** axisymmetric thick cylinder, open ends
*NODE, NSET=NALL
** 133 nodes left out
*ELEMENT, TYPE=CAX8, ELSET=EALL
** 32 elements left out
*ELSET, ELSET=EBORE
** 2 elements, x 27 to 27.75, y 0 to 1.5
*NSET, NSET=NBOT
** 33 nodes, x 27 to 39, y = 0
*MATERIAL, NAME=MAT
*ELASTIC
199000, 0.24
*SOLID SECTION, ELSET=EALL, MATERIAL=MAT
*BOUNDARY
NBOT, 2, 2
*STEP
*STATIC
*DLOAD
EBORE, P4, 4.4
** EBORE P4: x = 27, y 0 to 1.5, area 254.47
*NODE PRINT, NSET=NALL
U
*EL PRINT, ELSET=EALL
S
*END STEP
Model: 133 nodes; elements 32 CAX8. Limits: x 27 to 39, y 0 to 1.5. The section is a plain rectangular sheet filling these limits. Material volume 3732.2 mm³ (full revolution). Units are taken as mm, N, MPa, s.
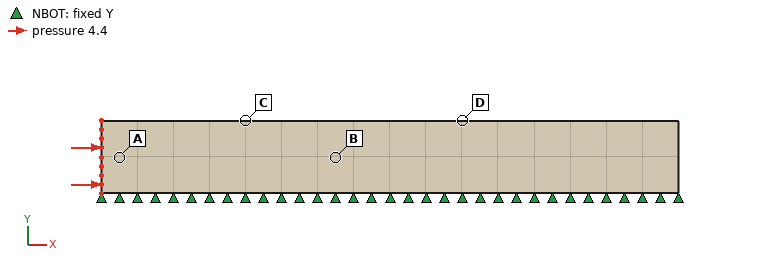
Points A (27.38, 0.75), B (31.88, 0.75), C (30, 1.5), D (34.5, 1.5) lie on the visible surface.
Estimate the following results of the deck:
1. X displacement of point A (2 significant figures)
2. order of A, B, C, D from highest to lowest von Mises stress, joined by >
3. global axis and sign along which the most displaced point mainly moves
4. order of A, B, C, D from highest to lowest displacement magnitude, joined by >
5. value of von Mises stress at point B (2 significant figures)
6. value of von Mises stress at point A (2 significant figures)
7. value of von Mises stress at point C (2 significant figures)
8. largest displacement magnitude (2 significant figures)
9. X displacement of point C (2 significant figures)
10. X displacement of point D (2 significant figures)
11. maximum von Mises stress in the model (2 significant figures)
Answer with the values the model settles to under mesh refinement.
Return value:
0.0018 mm
A > C > B > D
+X
A > C > B > D
11 MPa
15 MPa
13 MPa
0.0018 mm
0.0017 mm
0.0016 mm
15 MPa
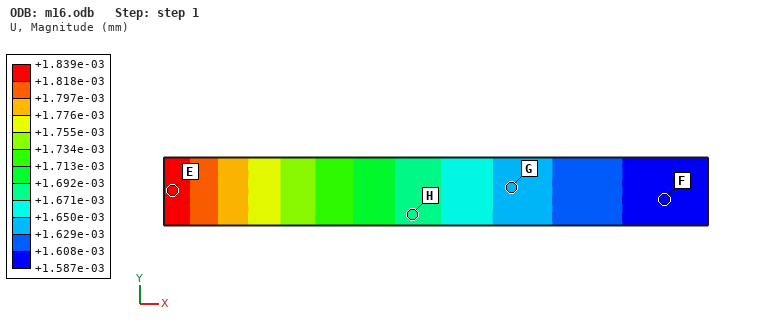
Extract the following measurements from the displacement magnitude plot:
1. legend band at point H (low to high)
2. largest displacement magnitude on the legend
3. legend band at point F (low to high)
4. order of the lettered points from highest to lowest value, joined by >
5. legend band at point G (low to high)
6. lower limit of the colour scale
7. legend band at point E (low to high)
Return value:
+1.671e-03 to +1.692e-03 mm
+1.839e-03 mm
+1.587e-03 to +1.608e-03 mm
E > H > G > F
+1.629e-03 to +1.650e-03 mm
+1.587e-03 mm
+1.818e-03 to +1.839e-03 mm
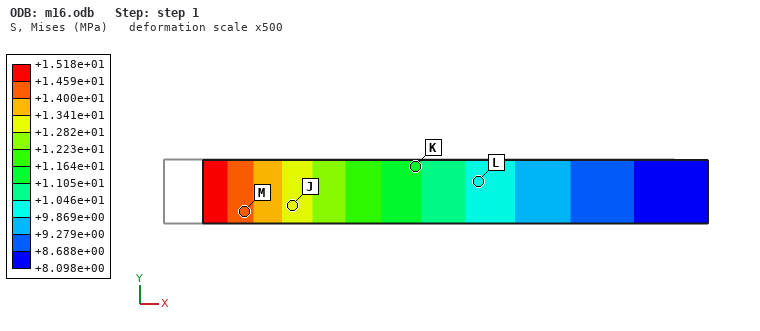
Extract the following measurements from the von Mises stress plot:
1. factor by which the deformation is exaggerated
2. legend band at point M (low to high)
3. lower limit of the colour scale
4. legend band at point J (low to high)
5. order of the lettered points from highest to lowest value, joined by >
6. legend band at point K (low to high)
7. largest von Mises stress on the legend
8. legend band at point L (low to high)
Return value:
500
+1.400e+01 to +1.459e+01 MPa
+8.098e+00 MPa
+1.282e+01 to +1.341e+01 MPa
M > J > K > L
+1.105e+01 to +1.164e+01 MPa
+1.518e+01 MPa
+9.869e+00 to +1.046e+01 MPa
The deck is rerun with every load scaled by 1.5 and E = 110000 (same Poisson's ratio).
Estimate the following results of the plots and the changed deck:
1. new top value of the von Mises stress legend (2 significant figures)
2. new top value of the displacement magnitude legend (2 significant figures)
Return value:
23 MPa
0.0050 mm
